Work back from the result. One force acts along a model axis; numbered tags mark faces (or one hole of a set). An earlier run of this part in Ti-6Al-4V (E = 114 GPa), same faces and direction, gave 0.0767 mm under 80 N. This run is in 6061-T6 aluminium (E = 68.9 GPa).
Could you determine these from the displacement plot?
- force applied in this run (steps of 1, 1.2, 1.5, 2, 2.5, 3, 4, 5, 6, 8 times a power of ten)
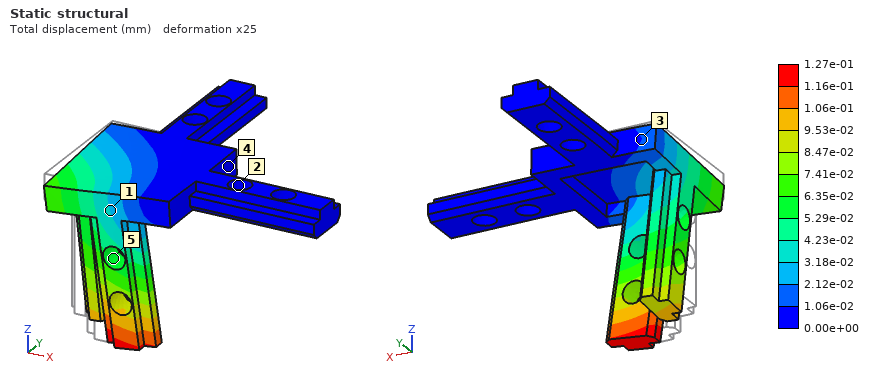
80 N
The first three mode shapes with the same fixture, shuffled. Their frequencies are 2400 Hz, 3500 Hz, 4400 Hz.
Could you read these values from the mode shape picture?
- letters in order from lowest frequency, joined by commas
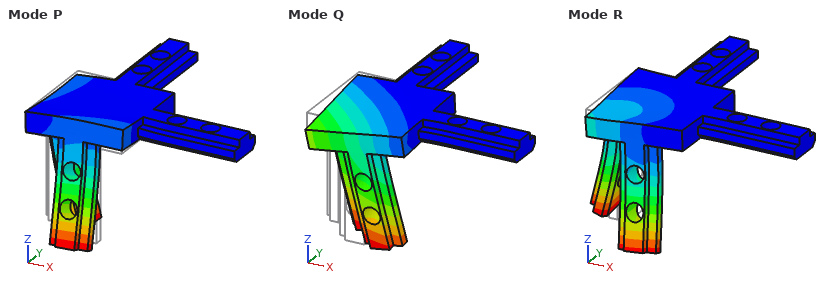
Q, P, R
